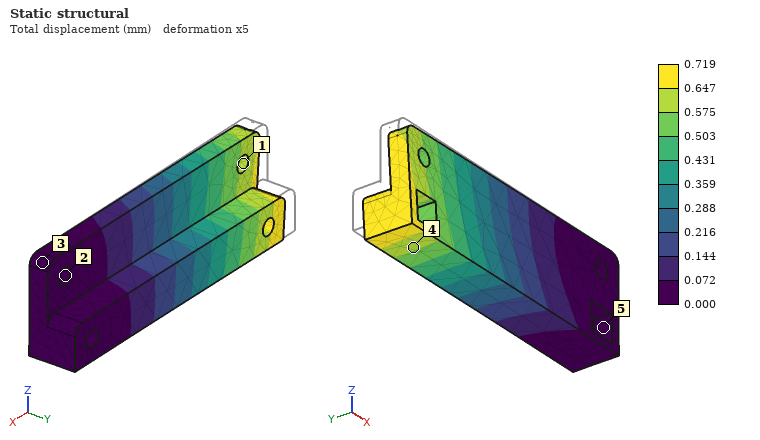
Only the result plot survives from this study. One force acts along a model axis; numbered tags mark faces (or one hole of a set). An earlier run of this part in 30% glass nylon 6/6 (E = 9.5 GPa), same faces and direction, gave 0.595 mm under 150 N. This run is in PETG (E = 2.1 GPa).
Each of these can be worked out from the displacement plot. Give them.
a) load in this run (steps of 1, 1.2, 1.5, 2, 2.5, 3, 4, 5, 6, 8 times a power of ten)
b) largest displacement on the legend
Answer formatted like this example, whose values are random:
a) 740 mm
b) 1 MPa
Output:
a) 40 N
b) 0.719 mm
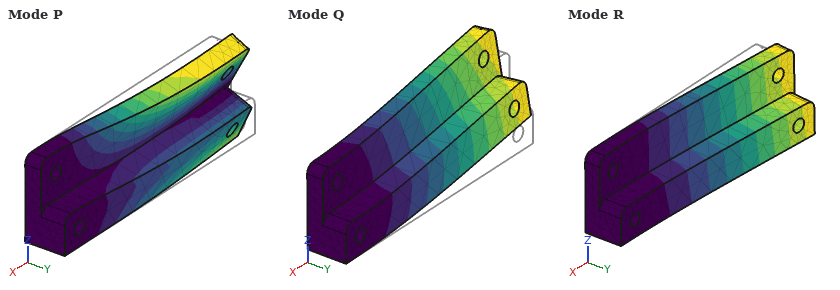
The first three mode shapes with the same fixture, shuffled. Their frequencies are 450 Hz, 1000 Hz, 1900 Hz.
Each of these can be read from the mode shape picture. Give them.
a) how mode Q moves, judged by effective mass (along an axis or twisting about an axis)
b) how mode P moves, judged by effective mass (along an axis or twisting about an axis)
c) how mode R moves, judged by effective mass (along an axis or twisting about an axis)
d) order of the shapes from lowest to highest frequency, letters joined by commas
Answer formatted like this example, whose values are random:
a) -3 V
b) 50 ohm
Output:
a) along Z
b) twisting about X
c) along Y
d) R, Q, P
